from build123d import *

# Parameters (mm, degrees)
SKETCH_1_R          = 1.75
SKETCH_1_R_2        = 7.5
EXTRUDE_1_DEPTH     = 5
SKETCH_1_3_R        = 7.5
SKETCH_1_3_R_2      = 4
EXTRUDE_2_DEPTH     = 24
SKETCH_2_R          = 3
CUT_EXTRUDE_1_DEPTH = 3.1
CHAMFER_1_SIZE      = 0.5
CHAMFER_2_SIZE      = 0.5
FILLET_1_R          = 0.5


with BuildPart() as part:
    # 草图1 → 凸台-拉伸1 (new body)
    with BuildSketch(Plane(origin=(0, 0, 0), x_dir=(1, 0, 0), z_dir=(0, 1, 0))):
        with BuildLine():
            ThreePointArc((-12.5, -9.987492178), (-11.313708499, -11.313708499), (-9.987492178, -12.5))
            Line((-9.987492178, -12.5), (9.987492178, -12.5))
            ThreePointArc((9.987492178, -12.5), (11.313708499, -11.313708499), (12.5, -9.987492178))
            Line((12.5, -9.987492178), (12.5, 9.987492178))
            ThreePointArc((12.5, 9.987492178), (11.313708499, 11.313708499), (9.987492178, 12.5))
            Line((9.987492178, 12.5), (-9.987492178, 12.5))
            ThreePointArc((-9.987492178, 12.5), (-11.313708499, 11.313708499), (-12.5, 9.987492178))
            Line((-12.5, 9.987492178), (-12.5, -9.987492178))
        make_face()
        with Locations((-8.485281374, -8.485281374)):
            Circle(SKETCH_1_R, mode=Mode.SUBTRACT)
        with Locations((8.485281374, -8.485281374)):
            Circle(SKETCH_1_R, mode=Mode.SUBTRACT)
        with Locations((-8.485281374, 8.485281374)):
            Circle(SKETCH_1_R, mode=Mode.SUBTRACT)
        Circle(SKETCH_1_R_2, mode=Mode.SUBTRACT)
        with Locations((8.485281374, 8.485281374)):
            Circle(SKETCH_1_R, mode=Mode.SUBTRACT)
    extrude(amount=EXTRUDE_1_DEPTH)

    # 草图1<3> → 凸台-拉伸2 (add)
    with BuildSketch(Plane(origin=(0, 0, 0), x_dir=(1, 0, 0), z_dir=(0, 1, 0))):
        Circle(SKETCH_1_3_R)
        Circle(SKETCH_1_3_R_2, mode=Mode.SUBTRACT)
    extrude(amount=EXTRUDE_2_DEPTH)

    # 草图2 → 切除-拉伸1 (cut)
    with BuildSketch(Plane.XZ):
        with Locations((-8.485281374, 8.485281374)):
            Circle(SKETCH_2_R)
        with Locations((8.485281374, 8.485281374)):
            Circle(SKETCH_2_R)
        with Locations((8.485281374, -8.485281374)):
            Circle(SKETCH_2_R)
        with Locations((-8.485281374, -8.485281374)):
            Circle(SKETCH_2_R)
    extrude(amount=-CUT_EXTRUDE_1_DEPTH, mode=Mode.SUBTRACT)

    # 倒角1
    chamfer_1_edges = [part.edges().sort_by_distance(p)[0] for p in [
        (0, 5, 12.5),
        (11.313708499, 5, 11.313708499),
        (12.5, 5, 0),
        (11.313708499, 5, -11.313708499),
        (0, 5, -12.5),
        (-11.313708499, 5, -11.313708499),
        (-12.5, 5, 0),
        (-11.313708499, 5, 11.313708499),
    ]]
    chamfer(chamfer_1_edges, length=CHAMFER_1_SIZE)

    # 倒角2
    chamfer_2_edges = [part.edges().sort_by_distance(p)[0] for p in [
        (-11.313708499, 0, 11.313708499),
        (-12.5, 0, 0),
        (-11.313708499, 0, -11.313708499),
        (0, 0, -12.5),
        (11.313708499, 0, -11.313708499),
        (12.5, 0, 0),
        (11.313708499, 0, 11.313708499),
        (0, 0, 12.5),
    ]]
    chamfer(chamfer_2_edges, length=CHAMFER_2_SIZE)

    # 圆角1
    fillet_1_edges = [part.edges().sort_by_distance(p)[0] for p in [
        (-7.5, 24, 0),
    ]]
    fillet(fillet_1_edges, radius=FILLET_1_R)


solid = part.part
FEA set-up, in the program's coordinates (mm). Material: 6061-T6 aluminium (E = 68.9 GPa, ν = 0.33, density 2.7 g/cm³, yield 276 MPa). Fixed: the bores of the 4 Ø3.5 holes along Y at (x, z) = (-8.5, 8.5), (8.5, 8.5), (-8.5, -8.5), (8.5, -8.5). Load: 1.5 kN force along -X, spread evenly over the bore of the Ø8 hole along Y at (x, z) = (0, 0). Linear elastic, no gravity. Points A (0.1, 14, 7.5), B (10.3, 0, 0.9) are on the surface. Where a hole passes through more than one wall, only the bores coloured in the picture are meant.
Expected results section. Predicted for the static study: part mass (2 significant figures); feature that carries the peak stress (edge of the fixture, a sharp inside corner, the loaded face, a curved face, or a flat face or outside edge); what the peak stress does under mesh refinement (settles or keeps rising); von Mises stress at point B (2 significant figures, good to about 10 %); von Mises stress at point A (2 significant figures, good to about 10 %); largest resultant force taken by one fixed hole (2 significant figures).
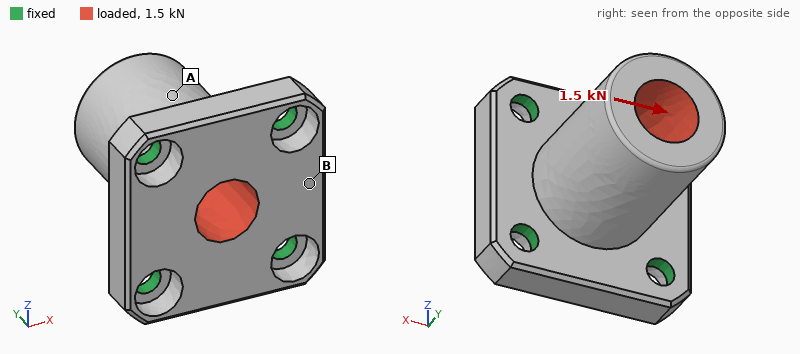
13 g
edge of the fixture
keeps rising
27 MPa
12 MPa
530 N
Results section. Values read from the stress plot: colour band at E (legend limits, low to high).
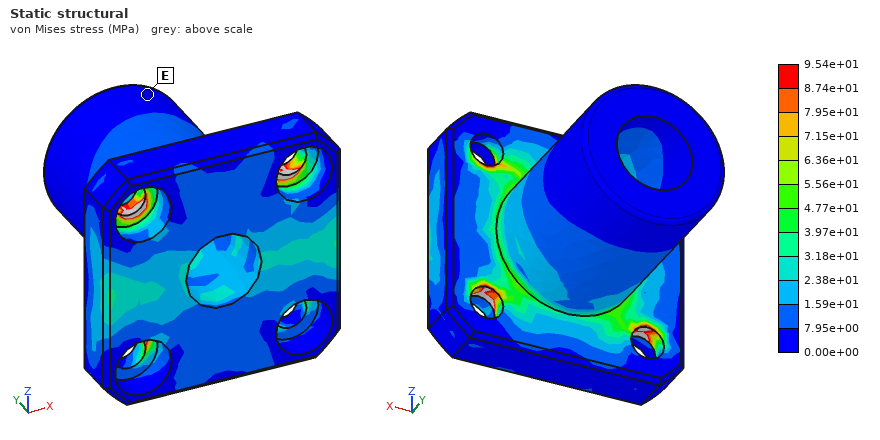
0.00e+00 to 7.95e+00 MPa
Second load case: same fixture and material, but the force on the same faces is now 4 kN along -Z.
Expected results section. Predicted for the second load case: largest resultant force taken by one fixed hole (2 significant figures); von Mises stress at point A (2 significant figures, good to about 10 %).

1.4 kN
25 MPa
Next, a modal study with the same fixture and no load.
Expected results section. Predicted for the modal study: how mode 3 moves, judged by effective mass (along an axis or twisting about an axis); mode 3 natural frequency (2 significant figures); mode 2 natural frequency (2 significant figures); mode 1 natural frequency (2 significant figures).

along Y
27 kHz
14 kHz
14 kHz
